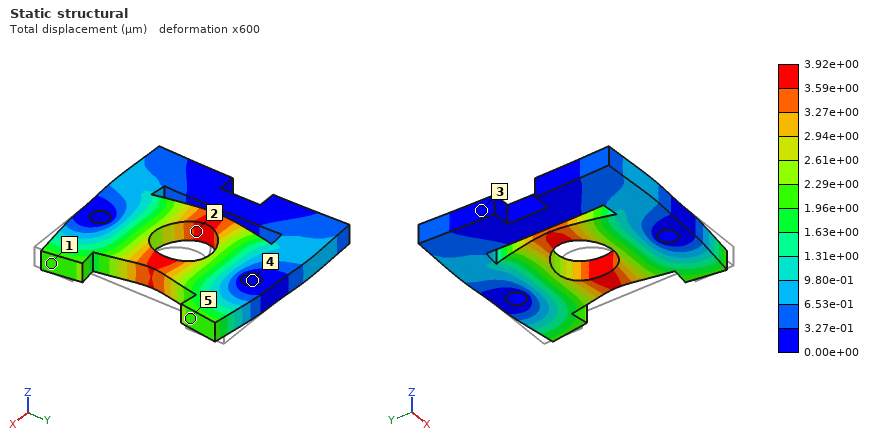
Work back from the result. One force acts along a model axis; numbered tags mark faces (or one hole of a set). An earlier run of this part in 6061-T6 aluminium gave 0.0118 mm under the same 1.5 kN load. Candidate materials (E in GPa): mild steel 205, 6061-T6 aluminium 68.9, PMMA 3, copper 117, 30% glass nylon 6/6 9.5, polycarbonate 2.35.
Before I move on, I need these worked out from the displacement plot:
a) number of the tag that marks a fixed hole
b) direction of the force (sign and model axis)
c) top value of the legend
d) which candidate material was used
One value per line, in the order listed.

4
-X
3.92e+00 µm
mild steel
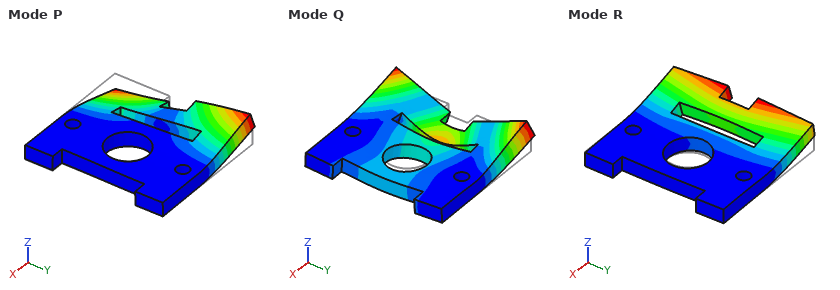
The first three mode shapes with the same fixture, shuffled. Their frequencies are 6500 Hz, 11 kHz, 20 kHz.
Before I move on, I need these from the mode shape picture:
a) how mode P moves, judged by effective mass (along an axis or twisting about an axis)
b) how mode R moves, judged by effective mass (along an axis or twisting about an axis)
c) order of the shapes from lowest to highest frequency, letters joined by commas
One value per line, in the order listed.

twisting about X
along Z
R, P, Q
